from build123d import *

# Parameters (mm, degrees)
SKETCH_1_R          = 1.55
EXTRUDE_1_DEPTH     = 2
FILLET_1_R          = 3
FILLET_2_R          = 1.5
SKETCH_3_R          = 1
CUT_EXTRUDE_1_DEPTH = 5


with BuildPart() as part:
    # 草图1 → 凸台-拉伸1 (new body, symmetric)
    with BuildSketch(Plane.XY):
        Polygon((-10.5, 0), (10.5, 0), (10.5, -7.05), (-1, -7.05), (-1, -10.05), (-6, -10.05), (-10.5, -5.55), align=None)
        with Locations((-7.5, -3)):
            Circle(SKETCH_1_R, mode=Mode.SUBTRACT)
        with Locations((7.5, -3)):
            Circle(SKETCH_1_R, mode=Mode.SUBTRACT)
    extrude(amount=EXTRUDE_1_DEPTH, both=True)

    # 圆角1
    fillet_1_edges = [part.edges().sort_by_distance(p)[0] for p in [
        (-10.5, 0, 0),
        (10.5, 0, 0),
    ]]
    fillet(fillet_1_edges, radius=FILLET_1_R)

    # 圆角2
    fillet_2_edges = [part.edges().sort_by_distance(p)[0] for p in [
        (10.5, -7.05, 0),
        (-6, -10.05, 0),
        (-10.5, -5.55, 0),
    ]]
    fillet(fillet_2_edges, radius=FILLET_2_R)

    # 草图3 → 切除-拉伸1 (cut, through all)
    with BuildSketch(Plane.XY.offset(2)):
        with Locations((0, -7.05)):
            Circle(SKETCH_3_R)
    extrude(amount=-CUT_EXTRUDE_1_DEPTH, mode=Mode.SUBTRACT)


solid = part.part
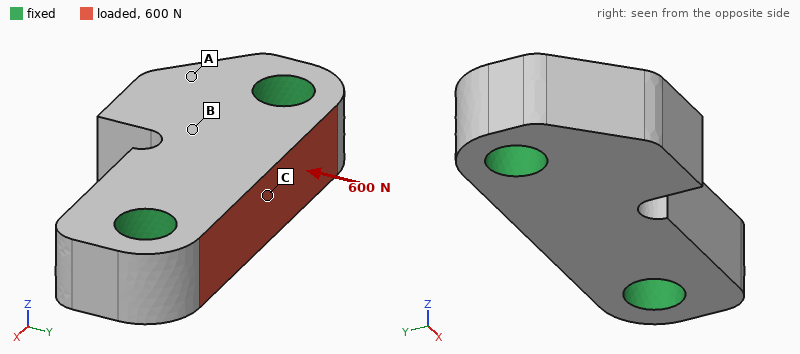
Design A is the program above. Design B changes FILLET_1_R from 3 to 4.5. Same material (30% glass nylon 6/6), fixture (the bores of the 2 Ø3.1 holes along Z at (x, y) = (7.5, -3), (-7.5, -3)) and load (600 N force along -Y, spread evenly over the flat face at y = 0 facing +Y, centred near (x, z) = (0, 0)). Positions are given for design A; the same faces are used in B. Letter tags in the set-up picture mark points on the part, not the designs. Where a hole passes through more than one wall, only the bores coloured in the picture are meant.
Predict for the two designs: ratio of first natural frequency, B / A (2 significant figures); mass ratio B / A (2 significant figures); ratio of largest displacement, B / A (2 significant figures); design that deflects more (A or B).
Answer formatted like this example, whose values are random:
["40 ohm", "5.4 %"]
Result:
["1.00", "0.97", "1.2", "B"]
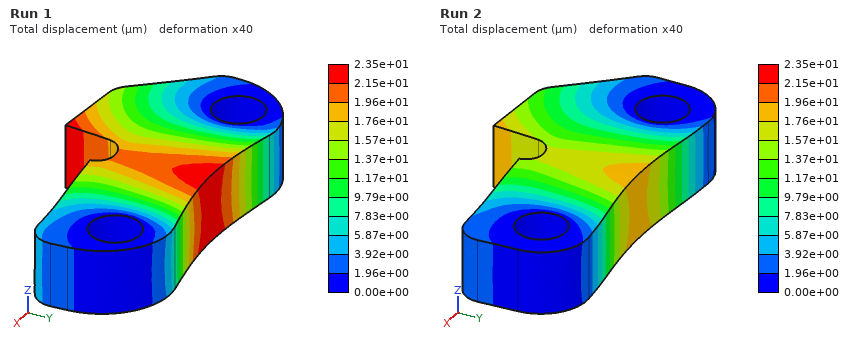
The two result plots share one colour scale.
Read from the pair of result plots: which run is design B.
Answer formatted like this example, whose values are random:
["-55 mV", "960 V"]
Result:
["Run 1"]
